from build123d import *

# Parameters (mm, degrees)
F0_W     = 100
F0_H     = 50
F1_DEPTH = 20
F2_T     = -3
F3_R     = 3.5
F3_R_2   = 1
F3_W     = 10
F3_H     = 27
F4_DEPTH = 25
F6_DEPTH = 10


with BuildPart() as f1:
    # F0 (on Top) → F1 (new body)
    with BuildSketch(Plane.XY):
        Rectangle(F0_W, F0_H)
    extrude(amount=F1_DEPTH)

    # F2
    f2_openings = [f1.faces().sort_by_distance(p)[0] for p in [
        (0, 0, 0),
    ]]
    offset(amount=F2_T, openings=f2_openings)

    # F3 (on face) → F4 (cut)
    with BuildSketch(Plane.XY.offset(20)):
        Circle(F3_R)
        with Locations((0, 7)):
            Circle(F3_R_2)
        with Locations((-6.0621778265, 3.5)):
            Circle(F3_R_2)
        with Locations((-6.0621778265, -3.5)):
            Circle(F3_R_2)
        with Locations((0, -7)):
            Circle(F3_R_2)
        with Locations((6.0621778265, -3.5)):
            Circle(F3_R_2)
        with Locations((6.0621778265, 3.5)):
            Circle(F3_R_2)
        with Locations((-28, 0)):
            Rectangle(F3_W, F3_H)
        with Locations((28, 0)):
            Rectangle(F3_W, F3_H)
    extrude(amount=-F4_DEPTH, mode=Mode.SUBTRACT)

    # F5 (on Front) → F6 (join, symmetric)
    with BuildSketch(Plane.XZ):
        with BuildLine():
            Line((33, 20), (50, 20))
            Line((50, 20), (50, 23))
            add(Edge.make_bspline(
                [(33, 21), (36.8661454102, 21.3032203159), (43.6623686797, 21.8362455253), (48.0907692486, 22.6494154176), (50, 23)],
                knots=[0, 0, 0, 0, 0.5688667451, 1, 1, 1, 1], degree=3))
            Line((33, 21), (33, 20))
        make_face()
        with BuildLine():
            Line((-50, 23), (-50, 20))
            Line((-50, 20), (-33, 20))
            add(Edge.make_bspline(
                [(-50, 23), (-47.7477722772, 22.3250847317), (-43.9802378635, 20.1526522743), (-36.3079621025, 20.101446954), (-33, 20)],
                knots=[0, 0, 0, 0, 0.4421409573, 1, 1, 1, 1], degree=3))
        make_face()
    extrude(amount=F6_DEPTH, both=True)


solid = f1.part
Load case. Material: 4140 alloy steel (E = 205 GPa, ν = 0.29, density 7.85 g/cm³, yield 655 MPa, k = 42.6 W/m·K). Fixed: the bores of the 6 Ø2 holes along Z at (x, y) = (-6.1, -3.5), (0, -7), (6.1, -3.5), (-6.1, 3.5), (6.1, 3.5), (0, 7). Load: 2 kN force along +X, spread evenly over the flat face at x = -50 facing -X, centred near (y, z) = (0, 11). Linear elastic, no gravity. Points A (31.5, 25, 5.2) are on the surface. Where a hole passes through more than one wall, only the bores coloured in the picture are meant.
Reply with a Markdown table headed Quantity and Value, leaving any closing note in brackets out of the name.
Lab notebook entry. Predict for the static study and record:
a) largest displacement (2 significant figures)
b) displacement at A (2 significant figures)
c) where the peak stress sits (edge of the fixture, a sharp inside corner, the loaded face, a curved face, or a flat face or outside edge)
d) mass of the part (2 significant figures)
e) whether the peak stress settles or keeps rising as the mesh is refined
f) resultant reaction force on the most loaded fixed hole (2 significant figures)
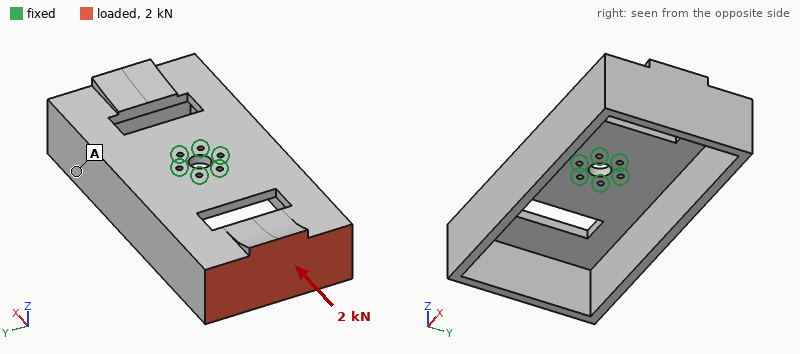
| Quantity | Value |
|---|---|
| largest displacement | 0.16 mm |
| displacement at A | 0.083 mm |
| where the peak stress sits | edge of the fixture |
| mass of the part | 230 g |
| whether the peak stress settles or keeps rising as the mesh is refined | keeps rising |
| resultant reaction force on the most loaded fixed hole | 480 N |
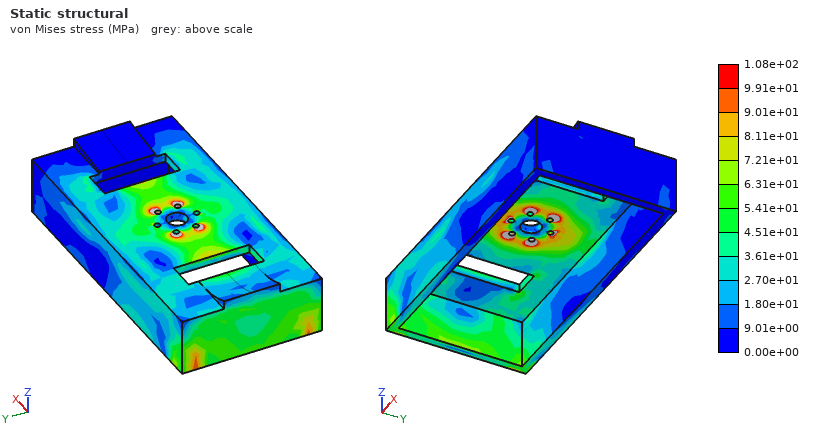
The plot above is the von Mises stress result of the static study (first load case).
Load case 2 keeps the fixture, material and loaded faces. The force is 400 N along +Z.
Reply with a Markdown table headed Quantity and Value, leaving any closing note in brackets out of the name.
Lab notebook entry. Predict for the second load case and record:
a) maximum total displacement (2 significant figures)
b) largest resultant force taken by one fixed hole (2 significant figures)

| Quantity | Value |
|---|---|
| maximum total displacement | 0.18 mm |
| largest resultant force taken by one fixed hole | 460 N |
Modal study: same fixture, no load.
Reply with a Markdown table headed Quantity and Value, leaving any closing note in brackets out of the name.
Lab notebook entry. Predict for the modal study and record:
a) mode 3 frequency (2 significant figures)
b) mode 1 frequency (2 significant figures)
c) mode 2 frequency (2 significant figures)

| Quantity | Value |
|---|---|
| mode 3 frequency | 1600 Hz |
| mode 1 frequency | 800 Hz |
| mode 2 frequency | 1600 Hz |
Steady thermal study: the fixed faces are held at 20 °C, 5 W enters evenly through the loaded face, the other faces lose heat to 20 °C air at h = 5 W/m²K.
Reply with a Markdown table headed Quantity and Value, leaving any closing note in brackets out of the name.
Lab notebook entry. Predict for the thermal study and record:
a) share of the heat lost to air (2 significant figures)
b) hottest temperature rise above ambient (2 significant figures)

| Quantity | Value |
|---|---|
| share of the heat lost to air | 20 % |
| hottest temperature rise above ambient | 34 K |
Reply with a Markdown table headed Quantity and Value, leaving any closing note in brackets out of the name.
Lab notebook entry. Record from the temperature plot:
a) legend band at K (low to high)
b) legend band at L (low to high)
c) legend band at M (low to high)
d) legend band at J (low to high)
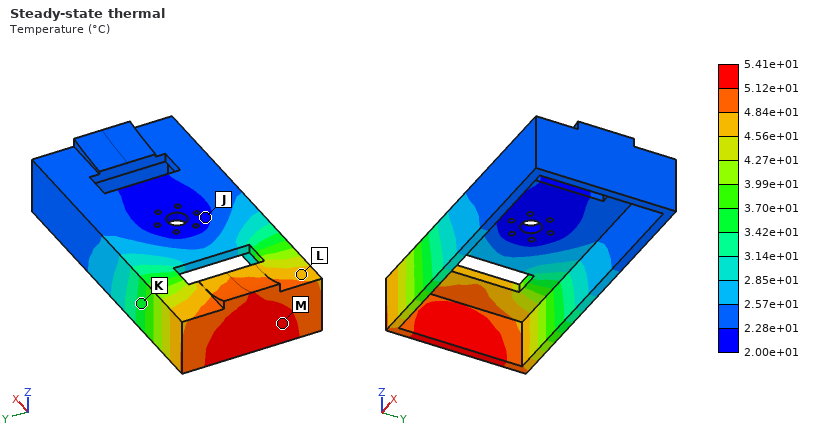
| Quantity | Value |
|---|---|
| legend band at K | 3.42e+01 to 3.70e+01 °C |
| legend band at L | 4.56e+01 to 4.84e+01 °C |
| legend band at M | 5.12e+01 to 5.41e+01 °C |
| legend band at J | 2.00e+01 to 2.28e+01 °C |
